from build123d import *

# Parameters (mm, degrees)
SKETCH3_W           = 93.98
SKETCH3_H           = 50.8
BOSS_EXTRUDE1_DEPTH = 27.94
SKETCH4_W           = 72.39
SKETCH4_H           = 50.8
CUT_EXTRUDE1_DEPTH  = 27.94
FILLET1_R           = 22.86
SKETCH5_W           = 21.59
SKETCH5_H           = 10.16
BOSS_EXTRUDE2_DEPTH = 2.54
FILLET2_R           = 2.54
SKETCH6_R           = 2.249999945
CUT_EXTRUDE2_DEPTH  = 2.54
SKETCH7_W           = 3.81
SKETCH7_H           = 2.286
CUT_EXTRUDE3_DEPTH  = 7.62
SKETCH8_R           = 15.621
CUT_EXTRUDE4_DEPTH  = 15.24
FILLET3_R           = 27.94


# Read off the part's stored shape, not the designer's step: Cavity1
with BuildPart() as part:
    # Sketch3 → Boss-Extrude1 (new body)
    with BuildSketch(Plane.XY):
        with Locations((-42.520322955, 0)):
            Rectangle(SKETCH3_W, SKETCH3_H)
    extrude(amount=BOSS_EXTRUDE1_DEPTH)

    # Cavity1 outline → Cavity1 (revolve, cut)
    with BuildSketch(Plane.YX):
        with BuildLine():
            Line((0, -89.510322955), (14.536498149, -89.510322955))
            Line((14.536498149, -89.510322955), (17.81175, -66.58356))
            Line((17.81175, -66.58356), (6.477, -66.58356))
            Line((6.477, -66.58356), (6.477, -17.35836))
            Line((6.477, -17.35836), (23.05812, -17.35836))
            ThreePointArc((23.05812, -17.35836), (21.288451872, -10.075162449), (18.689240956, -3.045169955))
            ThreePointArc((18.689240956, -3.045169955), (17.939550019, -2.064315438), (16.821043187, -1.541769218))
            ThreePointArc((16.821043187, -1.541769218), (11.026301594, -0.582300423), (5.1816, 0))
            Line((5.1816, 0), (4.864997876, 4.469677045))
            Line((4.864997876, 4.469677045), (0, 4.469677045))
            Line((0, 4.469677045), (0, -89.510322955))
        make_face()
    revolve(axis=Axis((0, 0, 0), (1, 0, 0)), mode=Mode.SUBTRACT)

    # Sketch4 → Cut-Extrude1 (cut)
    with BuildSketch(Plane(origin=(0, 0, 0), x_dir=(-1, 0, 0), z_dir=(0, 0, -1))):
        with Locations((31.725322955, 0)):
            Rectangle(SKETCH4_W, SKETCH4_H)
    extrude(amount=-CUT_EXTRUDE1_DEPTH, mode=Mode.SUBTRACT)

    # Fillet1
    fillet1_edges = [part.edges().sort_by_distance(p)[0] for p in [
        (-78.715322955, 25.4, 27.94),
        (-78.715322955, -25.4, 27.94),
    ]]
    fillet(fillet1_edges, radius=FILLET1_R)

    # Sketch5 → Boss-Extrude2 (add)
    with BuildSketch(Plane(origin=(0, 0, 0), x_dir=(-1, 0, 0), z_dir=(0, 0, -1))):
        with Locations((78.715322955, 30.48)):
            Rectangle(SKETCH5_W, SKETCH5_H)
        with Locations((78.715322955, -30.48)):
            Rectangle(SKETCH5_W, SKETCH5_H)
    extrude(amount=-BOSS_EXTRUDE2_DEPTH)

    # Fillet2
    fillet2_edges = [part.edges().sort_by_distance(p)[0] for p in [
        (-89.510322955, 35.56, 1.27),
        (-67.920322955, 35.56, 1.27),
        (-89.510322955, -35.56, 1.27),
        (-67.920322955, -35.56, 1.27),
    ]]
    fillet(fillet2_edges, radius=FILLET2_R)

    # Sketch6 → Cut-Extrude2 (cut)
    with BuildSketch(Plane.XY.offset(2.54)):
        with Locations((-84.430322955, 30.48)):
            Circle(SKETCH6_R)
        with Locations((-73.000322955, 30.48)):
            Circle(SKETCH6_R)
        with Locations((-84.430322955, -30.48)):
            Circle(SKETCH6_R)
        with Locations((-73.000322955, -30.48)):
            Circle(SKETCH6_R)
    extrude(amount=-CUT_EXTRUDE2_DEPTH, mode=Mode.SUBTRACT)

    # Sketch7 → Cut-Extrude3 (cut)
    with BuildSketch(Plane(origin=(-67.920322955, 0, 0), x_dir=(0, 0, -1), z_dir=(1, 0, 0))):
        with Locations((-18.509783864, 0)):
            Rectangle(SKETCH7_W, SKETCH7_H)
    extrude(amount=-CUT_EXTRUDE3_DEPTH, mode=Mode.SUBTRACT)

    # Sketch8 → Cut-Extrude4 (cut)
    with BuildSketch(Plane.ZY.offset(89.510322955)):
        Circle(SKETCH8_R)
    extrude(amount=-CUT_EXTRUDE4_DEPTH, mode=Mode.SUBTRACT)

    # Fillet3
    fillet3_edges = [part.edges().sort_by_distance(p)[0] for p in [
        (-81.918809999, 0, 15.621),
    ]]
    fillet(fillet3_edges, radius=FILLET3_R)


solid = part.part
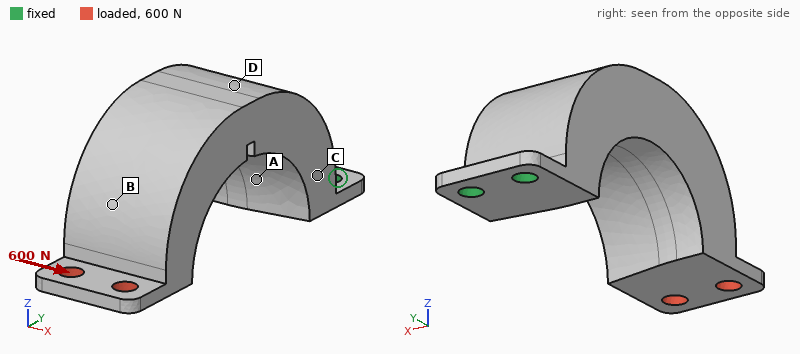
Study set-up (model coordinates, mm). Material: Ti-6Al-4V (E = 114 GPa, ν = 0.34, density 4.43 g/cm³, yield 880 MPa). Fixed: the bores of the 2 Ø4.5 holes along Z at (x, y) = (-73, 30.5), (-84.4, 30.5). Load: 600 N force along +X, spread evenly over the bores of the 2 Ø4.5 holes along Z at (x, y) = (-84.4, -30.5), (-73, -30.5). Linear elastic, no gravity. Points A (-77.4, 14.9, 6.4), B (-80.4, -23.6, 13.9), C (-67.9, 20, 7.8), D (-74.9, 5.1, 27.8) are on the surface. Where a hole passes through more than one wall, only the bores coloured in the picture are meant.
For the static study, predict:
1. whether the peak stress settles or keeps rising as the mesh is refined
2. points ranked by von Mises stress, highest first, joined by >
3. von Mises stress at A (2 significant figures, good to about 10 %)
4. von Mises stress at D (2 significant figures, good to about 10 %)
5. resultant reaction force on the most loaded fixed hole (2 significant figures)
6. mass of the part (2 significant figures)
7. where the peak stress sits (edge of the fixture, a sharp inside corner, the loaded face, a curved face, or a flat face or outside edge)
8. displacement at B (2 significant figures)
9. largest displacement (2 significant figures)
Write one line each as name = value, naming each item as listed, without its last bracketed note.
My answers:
whether the peak stress settles or keeps rising as the mesh is refined = keeps rising
points ranked by von Mises stress, highest first, joined by > = A > C > D > B
von Mises stress at A = 100 MPa
von Mises stress at D = 30 MPa
resultant reaction force on the most loaded fixed hole = 2.6 kN
mass of the part = 78 g
where the peak stress sits = edge of the fixture
displacement at B = 0.16 mm
largest displacement = 0.25 mm
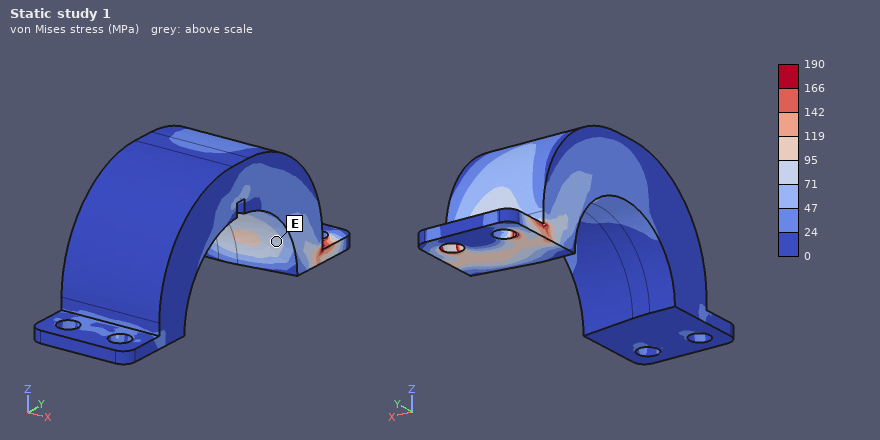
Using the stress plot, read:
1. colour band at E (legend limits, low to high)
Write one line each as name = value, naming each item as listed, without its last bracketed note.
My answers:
colour band at E = 71 to 95 MPa
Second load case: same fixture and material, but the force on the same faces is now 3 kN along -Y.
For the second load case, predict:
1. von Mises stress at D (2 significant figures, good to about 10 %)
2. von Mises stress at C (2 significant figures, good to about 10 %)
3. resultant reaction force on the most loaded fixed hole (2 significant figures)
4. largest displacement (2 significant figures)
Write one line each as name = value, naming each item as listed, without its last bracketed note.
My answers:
von Mises stress at D = 88 MPa
von Mises stress at C = 38 MPa
resultant reaction force on the most loaded fixed hole = 1.5 kN
largest displacement = 0.37 mm
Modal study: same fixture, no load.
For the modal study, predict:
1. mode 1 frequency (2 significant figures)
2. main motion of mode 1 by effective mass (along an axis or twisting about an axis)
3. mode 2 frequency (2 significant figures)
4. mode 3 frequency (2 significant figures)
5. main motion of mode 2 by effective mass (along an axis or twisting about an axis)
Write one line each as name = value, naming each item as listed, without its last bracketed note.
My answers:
mode 1 frequency = 430 Hz
main motion of mode 1 by effective mass = along Z
mode 2 frequency = 1900 Hz
mode 3 frequency = 3200 Hz
main motion of mode 2 by effective mass = along X
